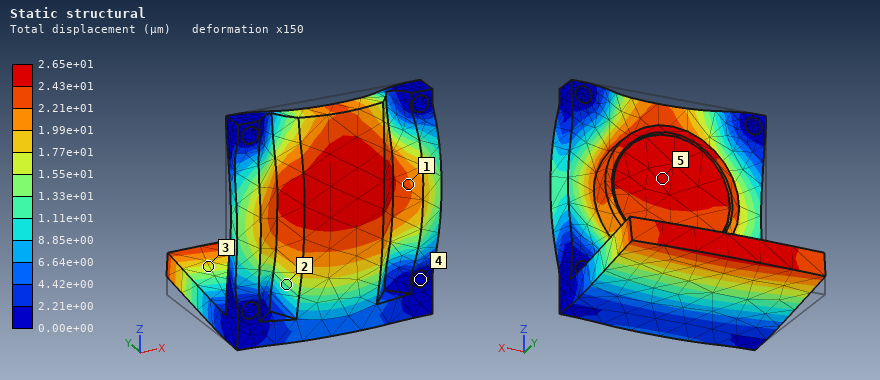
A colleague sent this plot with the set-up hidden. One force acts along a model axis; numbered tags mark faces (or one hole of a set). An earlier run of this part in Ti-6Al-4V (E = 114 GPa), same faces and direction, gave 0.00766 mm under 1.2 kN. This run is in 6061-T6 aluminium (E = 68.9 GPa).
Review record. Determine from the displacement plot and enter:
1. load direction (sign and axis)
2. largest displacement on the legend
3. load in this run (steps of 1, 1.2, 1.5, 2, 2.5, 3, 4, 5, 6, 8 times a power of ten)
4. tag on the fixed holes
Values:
-Y
2.65e+01 µm
2.5 kN
4
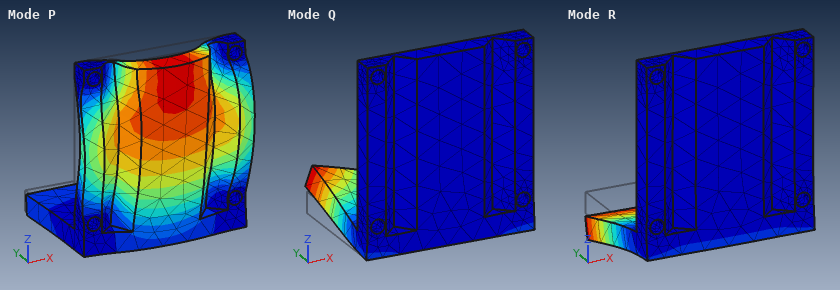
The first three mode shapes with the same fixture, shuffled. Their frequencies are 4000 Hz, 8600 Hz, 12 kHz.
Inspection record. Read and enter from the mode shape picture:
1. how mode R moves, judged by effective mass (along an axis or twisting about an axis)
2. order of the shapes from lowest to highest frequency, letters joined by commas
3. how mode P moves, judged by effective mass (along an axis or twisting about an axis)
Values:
along Z
R, Q, P
along Y
